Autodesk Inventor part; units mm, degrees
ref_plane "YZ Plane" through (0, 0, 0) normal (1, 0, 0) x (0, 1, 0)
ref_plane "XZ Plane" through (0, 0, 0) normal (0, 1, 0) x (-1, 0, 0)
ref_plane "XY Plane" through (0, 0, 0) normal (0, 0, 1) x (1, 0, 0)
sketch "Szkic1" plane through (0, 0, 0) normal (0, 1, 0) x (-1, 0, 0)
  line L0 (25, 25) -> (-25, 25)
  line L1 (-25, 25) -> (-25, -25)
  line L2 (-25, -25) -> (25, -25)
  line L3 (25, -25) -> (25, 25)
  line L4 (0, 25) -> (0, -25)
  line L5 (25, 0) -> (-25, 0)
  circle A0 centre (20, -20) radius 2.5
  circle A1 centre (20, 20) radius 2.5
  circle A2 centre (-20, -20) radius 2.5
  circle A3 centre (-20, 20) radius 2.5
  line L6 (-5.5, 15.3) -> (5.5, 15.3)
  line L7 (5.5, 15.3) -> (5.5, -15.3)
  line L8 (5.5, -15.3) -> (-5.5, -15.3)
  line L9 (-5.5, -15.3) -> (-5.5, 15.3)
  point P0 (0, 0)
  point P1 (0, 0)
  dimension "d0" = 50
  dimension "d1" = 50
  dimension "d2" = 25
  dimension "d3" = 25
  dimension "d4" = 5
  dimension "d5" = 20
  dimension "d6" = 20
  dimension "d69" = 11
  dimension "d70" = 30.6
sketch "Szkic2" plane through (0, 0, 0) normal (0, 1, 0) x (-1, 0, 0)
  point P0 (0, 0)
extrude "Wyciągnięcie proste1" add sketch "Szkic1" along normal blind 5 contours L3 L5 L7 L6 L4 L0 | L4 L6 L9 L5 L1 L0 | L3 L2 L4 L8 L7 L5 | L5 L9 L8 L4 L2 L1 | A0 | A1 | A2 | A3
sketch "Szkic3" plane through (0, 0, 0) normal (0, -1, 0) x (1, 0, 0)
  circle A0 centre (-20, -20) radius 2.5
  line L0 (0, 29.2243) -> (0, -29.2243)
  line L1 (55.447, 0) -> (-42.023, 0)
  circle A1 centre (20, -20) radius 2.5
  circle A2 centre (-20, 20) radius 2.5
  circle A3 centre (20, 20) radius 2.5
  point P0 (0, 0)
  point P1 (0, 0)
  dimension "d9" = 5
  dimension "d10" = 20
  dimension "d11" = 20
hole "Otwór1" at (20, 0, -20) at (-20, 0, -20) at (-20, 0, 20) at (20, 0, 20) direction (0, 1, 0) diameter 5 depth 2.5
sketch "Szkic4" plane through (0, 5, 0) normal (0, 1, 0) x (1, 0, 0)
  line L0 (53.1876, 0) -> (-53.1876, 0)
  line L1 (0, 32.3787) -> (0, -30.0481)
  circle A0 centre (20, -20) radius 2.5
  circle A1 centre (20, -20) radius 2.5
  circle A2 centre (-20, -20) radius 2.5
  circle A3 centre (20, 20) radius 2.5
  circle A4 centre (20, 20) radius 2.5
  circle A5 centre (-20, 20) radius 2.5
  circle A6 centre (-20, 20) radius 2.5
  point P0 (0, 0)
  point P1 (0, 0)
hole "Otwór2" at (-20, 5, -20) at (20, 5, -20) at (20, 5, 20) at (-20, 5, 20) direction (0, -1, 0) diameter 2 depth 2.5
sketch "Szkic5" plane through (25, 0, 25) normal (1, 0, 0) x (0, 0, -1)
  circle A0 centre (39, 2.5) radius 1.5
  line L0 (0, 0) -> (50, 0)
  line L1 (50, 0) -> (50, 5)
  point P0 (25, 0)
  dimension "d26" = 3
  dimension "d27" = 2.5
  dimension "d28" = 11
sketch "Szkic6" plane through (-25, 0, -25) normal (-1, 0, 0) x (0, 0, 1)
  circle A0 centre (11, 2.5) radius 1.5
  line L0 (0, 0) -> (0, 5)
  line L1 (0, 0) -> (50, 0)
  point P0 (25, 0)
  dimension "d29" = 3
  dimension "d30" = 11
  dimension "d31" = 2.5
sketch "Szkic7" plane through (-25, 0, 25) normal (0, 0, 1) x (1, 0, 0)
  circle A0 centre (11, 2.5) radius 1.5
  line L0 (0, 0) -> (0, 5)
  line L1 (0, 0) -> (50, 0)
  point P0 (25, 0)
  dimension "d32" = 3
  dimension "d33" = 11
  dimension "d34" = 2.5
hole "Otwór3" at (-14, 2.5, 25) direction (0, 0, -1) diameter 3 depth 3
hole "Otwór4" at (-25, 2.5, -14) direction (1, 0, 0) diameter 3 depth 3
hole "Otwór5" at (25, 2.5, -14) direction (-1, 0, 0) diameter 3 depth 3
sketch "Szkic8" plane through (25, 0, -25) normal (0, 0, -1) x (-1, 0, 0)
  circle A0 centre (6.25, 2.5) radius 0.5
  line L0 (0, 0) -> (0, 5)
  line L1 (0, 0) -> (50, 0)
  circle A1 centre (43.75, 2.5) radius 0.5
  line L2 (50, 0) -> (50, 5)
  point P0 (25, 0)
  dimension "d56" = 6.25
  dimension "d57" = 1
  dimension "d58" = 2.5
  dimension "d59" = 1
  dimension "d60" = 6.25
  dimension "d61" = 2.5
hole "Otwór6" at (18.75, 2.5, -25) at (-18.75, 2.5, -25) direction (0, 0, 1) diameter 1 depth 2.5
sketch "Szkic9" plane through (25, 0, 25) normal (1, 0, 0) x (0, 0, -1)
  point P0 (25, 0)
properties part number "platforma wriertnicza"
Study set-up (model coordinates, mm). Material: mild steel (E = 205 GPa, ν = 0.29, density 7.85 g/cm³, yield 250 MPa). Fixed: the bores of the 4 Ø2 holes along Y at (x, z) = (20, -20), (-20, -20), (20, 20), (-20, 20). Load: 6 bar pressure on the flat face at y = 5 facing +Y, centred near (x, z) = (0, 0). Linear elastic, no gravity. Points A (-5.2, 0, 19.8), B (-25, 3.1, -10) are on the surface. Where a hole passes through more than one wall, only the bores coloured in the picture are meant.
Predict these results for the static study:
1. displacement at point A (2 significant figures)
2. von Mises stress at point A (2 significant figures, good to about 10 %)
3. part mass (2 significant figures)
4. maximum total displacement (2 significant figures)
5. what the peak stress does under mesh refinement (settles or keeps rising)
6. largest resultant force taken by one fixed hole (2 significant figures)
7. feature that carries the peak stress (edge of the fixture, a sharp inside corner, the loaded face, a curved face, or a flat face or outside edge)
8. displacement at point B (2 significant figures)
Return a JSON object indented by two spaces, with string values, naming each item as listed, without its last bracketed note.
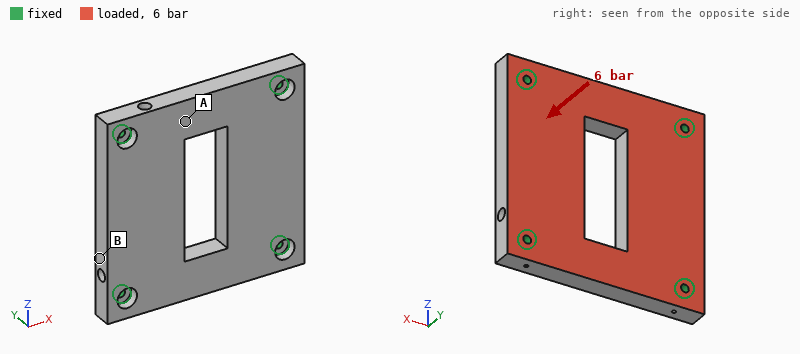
{
  "displacement at point A": "6.2 µm",
  "von Mises stress at point A": "23 MPa",
  "part mass": "83 g",
  "maximum total displacement": "12 µm",
  "what the peak stress does under mesh refinement": "keeps rising",
  "largest resultant force taken by one fixed hole": "410 N",
  "feature that carries the peak stress": "edge of the fixture",
  "displacement at point B": "1.9 µm"
}
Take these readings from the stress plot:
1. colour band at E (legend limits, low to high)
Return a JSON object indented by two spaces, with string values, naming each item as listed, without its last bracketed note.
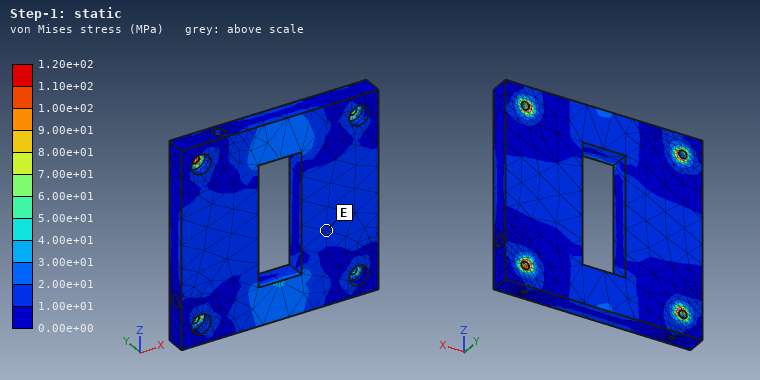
{
  "colour band at E": "1.00e+01 to 2.00e+01 MPa"
}
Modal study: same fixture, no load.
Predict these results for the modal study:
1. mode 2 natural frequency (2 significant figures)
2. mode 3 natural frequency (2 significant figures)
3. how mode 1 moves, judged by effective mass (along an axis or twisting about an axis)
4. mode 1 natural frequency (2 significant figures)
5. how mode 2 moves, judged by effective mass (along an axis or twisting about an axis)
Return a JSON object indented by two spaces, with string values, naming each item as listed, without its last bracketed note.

{
  "mode 2 natural frequency": "11 kHz",
  "mode 3 natural frequency": "12 kHz",
  "how mode 1 moves, judged by effective mass": "along Y",
  "mode 1 natural frequency": "7500 Hz",
  "how mode 2 moves, judged by effective mass": "twisting about Z"
}
